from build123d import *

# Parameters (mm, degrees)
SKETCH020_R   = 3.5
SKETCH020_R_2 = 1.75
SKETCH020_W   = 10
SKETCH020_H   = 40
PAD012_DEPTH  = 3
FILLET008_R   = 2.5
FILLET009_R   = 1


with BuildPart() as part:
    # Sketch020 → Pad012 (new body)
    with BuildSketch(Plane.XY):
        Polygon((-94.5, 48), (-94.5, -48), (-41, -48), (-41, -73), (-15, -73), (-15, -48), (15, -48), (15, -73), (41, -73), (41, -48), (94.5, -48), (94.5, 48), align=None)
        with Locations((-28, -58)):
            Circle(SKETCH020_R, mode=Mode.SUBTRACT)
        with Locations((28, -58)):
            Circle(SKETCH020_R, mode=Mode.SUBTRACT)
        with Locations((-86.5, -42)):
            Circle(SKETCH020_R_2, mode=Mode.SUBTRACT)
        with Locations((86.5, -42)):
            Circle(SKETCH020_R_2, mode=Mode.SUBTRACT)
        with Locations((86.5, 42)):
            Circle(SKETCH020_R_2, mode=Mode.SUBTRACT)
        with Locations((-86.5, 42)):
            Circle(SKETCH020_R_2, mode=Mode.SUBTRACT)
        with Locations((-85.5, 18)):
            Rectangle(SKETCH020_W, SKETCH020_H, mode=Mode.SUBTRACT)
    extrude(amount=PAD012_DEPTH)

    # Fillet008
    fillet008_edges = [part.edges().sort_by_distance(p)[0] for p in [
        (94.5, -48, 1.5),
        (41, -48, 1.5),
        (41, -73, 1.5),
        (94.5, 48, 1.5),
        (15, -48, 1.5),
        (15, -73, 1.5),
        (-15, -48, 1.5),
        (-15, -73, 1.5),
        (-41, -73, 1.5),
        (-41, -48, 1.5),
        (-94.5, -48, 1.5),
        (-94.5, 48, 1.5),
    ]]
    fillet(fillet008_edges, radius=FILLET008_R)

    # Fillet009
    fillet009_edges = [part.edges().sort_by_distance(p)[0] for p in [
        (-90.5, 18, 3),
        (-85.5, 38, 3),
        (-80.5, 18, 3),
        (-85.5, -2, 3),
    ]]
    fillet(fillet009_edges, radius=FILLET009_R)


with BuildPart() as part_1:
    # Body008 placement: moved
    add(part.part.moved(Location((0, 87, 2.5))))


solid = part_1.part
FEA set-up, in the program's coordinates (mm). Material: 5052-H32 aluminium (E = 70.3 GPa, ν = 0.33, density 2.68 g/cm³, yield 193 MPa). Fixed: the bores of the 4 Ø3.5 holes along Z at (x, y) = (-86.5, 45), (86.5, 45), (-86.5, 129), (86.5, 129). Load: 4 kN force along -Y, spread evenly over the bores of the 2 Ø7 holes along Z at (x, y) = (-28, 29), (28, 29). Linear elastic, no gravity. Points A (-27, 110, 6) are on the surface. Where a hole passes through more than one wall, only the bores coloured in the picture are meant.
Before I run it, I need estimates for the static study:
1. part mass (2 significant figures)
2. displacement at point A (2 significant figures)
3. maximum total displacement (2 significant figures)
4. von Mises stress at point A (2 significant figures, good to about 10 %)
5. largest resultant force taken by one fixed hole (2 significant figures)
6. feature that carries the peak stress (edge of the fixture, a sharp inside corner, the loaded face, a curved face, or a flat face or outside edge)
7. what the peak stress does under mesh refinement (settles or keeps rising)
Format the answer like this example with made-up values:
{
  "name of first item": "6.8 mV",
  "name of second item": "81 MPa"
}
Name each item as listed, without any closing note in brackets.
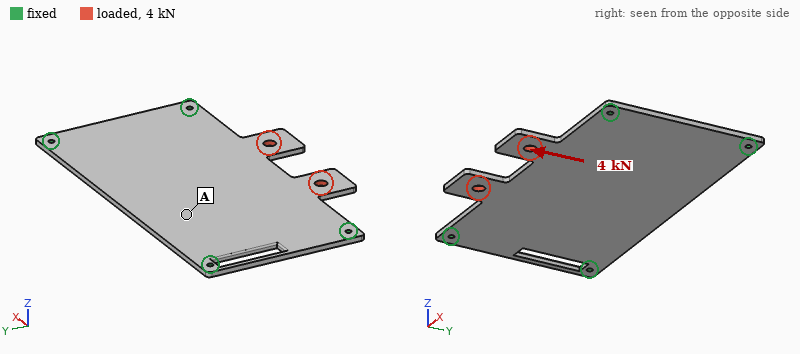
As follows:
{
  "part mass": "150 g",
  "displacement at point A": "26 µm",
  "maximum total displacement": "42 µm",
  "von Mises stress at point A": "9.0 MPa",
  "largest resultant force taken by one fixed hole": "1.4 kN",
  "feature that carries the peak stress": "a sharp inside corner",
  "what the peak stress does under mesh refinement": "keeps rising"
}
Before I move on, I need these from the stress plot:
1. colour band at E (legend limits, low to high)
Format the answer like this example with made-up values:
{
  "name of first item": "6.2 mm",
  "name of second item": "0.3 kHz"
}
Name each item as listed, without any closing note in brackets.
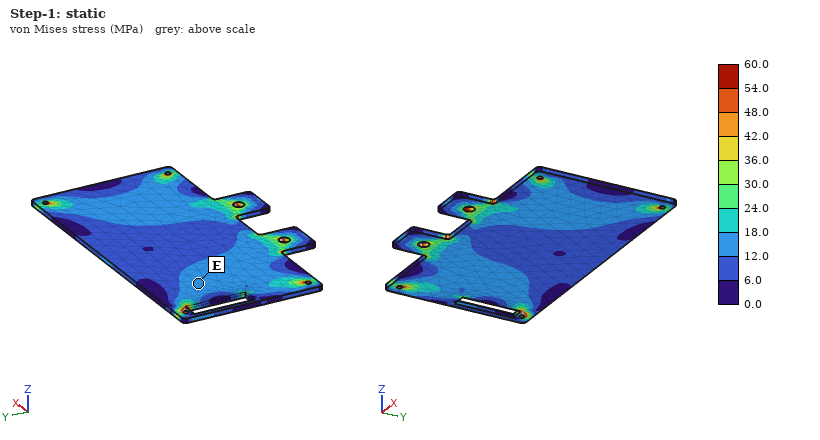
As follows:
{
  "colour band at E": "12.0 to 18.0 MPa"
}
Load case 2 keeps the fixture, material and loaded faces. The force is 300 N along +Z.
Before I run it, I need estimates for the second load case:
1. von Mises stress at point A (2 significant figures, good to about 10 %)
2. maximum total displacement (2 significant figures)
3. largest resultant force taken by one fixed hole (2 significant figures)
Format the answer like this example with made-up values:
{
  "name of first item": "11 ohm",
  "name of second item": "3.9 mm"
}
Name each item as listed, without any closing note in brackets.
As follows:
{
  "von Mises stress at point A": "17 MPa",
  "maximum total displacement": "1.8 mm",
  "largest resultant force taken by one fixed hole": "180 N"
}
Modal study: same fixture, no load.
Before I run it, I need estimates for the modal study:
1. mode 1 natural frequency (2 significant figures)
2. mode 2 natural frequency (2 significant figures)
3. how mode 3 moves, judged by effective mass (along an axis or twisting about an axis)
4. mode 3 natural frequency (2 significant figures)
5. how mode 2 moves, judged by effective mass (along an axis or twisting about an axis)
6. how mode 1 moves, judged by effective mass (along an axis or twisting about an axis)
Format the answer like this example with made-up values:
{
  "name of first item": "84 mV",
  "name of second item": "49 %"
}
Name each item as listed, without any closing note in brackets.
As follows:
{
  "mode 1 natural frequency": "400 Hz",
  "mode 2 natural frequency": "640 Hz",
  "how mode 3 moves, judged by effective mass": "twisting about Y",
  "mode 3 natural frequency": "1100 Hz",
  "how mode 2 moves, judged by effective mass": "twisting about X",
  "how mode 1 moves, judged by effective mass": "along Z"
}
